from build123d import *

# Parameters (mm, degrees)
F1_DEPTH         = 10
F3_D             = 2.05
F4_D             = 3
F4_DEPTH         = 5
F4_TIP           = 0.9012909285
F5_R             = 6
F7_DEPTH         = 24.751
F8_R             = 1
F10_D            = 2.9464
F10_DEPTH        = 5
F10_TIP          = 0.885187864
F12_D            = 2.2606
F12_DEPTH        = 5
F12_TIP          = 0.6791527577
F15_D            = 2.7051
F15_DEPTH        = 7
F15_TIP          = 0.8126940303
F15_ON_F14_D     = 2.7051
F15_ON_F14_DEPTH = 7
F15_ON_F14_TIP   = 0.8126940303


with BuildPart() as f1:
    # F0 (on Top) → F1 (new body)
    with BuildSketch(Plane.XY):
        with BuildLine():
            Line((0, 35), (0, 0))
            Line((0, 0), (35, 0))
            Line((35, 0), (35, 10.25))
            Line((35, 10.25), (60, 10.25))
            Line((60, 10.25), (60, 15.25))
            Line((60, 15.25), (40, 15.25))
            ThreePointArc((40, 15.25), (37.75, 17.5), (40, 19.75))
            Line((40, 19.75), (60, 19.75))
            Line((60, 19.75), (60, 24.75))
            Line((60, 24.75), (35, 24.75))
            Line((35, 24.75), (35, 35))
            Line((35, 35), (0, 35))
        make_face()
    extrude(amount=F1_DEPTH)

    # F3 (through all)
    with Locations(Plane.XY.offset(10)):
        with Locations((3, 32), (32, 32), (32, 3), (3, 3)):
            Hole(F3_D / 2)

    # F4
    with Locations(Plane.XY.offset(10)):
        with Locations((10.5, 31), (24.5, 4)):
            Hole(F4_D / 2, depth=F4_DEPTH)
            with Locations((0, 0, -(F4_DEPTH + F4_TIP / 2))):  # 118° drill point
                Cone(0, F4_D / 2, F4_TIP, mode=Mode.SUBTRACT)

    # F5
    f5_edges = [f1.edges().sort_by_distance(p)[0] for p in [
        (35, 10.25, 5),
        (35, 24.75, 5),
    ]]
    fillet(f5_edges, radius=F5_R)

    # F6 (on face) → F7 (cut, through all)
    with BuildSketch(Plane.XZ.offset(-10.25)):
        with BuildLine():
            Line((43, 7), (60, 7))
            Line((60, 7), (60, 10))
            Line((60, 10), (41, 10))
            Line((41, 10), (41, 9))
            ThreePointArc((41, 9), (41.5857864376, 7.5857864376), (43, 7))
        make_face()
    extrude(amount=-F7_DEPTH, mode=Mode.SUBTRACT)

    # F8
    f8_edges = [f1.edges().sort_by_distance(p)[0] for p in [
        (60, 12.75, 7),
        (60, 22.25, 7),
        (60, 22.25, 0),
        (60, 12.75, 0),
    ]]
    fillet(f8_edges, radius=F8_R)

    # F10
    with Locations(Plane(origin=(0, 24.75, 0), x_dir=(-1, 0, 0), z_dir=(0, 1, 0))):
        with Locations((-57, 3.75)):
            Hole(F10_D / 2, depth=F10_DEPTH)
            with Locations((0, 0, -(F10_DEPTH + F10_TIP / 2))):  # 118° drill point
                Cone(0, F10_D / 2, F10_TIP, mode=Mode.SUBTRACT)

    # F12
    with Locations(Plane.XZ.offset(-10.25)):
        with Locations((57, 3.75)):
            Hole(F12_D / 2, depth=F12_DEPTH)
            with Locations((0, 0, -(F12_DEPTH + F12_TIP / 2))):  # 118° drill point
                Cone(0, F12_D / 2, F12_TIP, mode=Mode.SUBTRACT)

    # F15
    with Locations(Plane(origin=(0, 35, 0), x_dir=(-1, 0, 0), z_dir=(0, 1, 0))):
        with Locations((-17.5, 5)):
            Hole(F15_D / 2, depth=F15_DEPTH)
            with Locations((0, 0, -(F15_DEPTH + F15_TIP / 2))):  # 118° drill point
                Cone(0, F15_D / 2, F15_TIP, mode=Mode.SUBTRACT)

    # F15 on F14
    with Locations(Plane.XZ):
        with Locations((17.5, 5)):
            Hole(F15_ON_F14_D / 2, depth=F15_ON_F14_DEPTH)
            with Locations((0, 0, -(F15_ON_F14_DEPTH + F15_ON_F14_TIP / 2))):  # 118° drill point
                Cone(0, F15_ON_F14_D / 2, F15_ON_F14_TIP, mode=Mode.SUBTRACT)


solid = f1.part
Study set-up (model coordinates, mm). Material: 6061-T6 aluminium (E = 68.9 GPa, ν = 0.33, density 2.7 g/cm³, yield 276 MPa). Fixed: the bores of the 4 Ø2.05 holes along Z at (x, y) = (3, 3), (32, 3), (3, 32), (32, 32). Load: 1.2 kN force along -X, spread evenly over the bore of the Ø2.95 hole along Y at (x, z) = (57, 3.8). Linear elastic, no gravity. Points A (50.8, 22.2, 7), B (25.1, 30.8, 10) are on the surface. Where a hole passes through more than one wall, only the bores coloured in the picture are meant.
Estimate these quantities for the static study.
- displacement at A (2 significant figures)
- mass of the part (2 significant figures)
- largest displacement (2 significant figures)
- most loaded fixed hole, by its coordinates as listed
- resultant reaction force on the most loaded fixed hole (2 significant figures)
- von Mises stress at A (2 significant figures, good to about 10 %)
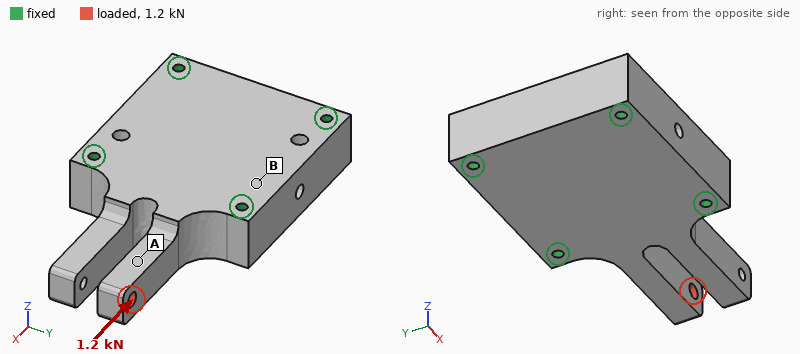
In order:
9.9 µm
38 g
16 µm
(32, 32)
540 N
44 MPa
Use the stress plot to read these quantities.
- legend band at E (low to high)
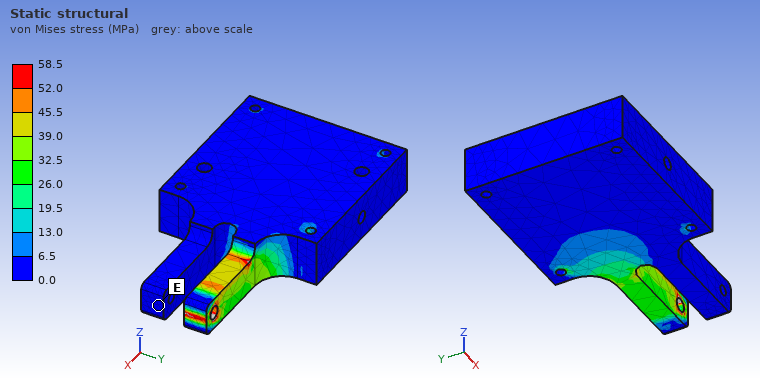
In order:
0.0 to 6.5 MPa
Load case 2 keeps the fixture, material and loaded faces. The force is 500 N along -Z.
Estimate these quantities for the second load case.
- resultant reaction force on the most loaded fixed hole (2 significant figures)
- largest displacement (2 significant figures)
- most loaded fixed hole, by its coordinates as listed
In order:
550 N
0.19 mm
(32, 32)
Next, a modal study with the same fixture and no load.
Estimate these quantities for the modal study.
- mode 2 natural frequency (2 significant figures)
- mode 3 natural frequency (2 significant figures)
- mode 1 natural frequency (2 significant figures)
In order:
8600 Hz
9300 Hz
8300 Hz
